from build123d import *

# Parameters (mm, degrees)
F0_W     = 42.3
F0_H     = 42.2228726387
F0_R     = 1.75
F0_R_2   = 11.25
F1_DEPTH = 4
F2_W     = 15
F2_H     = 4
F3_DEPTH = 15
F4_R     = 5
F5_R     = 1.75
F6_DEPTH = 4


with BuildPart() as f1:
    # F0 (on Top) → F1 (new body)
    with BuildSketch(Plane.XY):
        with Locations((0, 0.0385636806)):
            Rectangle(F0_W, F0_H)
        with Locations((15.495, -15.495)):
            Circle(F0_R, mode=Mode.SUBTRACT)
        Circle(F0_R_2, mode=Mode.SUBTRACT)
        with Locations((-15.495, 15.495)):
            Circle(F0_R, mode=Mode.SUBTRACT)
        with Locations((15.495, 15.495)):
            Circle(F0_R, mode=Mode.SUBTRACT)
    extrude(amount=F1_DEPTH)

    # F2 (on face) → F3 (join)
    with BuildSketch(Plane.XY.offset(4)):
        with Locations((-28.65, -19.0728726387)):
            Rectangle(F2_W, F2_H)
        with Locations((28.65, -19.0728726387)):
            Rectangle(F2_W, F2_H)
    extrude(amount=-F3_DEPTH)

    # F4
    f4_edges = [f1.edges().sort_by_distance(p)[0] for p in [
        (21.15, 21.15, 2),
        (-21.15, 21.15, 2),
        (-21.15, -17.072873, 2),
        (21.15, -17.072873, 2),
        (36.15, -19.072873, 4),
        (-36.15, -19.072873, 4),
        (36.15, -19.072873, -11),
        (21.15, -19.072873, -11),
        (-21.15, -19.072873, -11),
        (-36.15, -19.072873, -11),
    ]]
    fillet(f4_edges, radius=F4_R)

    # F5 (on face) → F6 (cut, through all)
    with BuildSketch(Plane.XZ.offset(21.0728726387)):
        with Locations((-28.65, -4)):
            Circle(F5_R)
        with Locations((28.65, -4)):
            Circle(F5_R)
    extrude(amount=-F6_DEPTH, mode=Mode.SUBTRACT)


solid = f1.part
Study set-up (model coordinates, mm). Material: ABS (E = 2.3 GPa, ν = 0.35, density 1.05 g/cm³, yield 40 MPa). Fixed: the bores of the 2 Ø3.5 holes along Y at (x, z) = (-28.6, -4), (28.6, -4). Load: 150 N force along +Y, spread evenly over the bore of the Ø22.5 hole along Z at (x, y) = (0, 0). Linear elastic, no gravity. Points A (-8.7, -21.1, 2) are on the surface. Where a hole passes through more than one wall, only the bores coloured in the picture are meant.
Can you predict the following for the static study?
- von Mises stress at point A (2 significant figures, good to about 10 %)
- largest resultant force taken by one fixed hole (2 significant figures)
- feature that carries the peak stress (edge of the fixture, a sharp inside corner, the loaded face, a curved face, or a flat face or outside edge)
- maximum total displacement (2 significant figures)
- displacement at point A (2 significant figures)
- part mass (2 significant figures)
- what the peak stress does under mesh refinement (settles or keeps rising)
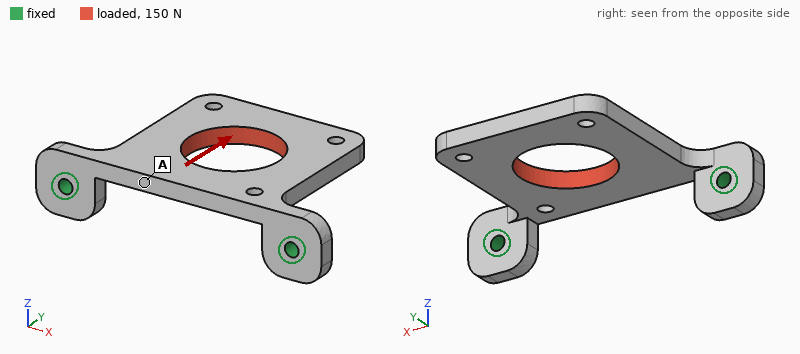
2.0 MPa
82 N
edge of the fixture
0.60 mm
0.16 mm
7.4 g
keeps rising
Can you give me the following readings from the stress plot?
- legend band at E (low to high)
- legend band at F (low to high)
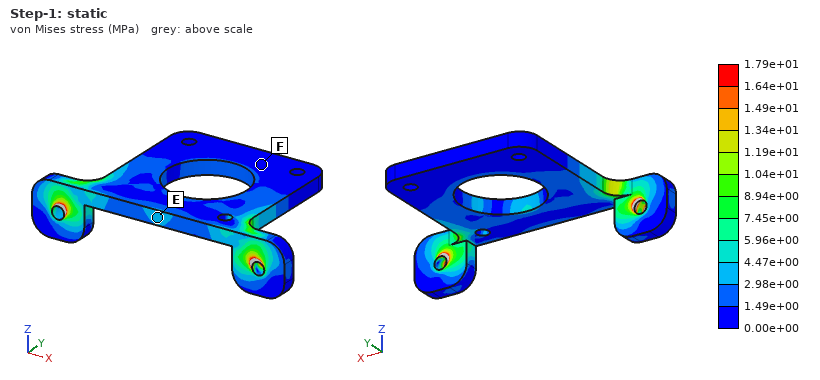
2.98e+00 to 4.47e+00 MPa
0.00e+00 to 1.49e+00 MPa
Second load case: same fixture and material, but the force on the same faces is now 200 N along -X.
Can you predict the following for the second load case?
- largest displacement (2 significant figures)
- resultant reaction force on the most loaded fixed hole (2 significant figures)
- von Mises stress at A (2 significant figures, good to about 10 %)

0.34 mm
130 N
3.1 MPa
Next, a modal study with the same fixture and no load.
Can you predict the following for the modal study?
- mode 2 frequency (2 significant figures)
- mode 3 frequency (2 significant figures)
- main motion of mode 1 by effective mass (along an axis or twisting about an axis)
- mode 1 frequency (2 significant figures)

1000 Hz
1900 Hz
along Z
310 Hz
